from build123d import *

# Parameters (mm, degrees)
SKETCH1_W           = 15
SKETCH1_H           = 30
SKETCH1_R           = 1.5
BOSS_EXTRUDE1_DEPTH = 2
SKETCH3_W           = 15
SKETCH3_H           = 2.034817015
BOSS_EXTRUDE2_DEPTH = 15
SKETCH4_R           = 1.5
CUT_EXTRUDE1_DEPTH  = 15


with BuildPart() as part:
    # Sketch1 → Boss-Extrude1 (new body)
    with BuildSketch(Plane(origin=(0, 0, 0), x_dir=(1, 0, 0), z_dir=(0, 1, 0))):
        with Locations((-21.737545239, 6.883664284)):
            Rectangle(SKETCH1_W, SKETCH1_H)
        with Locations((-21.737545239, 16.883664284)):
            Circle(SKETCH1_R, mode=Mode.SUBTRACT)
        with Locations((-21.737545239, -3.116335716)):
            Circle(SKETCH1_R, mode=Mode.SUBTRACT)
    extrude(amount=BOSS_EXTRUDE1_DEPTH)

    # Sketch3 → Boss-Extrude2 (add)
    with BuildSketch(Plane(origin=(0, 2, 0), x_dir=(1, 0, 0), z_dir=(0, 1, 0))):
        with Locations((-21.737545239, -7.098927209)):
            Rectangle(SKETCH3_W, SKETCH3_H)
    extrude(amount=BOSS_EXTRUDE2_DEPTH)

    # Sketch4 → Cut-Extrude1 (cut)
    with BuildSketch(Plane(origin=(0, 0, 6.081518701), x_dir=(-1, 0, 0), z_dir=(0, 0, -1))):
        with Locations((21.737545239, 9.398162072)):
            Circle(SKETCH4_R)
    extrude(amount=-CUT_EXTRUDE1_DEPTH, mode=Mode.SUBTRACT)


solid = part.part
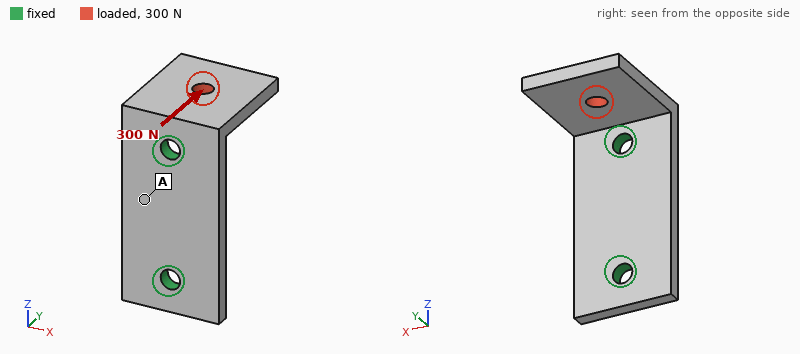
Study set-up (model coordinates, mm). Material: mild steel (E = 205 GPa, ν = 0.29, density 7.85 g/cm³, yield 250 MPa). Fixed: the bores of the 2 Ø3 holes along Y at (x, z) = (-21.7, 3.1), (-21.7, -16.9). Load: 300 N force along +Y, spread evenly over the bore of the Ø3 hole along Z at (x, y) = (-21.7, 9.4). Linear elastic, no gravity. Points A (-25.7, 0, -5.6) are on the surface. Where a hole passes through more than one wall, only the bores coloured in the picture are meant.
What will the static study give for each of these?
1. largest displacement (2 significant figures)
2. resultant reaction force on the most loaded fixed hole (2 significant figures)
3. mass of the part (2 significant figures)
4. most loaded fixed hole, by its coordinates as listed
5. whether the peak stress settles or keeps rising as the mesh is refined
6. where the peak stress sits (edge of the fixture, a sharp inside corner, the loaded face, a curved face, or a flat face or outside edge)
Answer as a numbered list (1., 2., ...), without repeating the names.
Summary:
1. 17 µm
2. 310 N
3. 10 g
4. (-21.7, 3.1)
5. keeps rising
6. edge of the fixture
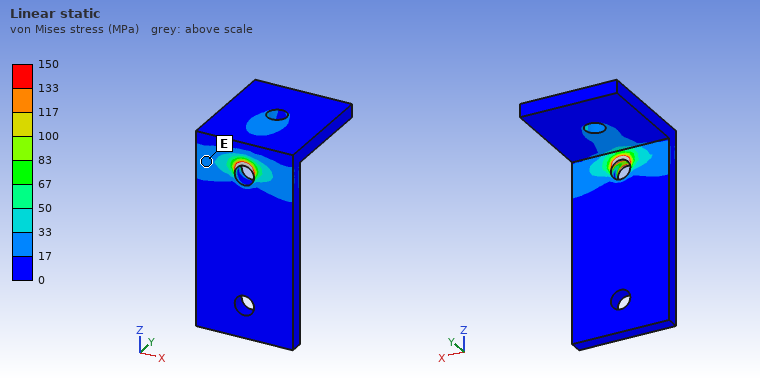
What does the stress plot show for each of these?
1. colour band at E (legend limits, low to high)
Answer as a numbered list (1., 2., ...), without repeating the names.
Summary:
1. 17 to 33 MPa
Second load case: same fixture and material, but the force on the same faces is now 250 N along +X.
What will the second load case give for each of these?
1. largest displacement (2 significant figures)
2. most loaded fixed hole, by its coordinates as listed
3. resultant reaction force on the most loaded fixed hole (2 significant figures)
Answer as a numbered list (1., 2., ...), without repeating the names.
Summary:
1. 36 µm
2. (-21.7, 3.1)
3. 280 N
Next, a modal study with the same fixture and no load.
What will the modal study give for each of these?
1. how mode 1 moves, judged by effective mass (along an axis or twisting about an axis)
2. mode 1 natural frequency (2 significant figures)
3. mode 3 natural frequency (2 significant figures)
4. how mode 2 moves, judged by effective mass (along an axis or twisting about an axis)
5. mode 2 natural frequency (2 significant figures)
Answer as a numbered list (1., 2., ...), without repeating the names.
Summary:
1. along Z
2. 4900 Hz
3. 15 kHz
4. along X
5. 8100 Hz
